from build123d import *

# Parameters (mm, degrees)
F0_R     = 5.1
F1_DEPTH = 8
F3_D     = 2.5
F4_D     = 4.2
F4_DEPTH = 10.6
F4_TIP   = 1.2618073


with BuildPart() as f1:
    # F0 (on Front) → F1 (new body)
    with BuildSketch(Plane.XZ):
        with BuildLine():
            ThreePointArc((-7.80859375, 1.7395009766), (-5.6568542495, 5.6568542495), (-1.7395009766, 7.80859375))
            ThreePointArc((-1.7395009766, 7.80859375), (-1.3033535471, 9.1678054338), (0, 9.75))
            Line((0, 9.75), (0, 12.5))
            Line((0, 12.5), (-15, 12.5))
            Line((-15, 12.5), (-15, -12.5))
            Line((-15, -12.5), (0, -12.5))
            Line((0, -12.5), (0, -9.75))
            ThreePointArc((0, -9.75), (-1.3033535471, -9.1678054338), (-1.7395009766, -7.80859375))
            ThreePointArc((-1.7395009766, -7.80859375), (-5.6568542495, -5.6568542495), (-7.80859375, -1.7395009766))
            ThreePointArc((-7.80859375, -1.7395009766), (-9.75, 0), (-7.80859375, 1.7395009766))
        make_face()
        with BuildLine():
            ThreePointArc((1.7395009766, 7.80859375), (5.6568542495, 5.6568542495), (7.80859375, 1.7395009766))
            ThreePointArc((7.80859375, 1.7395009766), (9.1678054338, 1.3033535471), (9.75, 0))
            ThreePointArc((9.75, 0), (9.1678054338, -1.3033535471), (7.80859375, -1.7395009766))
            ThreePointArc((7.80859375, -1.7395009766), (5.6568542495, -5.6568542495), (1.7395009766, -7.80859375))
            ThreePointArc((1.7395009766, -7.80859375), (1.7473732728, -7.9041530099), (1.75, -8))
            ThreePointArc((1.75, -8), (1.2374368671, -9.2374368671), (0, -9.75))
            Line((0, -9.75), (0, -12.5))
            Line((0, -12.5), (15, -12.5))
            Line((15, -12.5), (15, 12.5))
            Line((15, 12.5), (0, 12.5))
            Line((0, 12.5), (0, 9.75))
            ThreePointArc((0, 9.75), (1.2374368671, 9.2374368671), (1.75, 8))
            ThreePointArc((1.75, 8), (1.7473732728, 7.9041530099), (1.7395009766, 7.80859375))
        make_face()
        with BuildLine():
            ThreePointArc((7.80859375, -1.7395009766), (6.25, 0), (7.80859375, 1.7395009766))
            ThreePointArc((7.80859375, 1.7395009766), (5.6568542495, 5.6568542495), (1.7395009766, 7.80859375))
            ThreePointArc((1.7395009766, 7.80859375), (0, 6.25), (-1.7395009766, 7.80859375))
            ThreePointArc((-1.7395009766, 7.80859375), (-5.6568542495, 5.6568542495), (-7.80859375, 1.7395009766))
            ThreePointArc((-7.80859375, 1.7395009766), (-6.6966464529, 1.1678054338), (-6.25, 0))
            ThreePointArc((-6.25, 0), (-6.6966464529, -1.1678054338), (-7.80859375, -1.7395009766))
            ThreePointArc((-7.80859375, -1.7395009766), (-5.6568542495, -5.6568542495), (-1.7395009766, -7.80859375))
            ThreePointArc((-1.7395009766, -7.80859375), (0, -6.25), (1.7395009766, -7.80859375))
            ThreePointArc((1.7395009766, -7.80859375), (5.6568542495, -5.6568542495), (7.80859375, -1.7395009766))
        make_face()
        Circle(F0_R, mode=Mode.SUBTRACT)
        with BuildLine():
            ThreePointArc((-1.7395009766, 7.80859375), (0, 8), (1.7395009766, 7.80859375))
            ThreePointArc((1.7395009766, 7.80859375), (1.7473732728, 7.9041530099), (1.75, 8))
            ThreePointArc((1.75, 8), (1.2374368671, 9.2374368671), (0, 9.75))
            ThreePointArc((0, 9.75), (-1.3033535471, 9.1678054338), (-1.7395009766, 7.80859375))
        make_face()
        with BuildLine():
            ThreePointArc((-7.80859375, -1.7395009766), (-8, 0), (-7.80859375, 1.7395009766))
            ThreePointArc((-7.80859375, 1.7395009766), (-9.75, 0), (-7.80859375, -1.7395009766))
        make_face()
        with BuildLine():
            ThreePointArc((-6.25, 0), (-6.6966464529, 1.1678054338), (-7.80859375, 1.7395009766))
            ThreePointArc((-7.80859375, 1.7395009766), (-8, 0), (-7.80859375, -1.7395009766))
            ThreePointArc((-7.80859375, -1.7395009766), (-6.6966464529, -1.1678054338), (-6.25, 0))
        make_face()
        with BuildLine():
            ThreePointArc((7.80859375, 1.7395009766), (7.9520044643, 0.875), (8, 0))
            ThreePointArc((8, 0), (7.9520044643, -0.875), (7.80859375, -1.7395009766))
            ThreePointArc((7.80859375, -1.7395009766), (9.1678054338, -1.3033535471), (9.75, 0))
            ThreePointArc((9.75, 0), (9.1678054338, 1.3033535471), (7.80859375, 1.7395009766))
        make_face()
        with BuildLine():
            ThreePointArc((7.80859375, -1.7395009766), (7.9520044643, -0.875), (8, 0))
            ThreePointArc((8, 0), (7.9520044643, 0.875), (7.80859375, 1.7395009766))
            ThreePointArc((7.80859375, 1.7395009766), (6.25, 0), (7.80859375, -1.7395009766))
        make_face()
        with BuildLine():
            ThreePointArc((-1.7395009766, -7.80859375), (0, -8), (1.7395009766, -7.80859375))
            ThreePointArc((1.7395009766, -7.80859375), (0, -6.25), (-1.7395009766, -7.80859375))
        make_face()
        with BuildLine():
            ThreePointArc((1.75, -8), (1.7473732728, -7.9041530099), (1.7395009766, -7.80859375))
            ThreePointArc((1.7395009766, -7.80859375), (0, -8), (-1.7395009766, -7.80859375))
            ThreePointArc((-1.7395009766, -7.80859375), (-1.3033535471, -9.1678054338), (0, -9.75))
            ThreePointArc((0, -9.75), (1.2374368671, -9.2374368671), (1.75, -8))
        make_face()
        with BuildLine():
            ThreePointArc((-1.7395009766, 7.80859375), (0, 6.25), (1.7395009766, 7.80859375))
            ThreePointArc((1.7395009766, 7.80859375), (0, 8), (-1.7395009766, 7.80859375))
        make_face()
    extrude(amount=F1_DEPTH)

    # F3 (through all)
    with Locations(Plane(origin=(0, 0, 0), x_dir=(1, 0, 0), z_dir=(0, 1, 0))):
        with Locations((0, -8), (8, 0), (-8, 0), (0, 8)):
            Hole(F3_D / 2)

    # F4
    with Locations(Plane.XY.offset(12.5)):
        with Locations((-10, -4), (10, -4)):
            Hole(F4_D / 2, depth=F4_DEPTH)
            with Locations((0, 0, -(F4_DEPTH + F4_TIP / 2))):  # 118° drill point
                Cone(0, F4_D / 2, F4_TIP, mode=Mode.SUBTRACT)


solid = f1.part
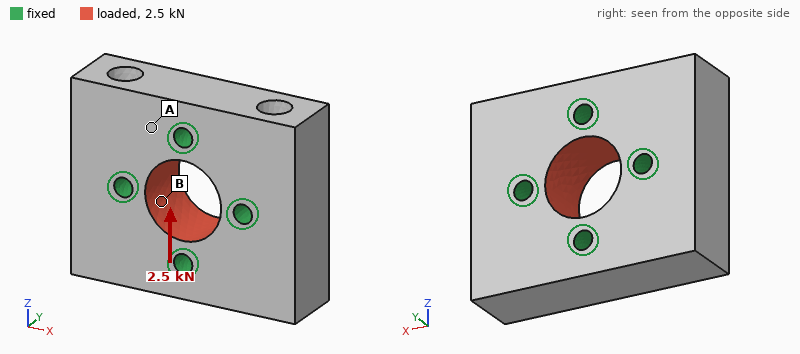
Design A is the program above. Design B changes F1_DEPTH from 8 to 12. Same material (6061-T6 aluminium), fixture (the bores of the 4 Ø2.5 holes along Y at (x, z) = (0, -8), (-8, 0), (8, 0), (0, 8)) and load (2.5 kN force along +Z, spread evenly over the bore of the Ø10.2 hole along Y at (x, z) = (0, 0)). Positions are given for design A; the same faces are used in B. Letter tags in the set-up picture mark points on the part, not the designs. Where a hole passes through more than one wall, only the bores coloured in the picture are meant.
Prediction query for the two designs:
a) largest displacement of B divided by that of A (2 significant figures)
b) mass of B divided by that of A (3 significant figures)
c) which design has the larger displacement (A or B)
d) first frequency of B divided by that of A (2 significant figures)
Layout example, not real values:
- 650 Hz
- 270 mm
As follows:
- 0.68
- 1.53
- A
- 1.2
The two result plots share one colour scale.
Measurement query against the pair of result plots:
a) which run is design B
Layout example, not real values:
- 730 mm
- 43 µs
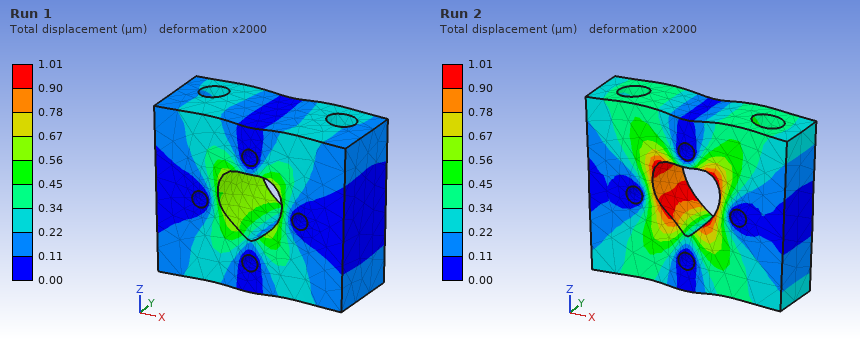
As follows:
- Run 1
